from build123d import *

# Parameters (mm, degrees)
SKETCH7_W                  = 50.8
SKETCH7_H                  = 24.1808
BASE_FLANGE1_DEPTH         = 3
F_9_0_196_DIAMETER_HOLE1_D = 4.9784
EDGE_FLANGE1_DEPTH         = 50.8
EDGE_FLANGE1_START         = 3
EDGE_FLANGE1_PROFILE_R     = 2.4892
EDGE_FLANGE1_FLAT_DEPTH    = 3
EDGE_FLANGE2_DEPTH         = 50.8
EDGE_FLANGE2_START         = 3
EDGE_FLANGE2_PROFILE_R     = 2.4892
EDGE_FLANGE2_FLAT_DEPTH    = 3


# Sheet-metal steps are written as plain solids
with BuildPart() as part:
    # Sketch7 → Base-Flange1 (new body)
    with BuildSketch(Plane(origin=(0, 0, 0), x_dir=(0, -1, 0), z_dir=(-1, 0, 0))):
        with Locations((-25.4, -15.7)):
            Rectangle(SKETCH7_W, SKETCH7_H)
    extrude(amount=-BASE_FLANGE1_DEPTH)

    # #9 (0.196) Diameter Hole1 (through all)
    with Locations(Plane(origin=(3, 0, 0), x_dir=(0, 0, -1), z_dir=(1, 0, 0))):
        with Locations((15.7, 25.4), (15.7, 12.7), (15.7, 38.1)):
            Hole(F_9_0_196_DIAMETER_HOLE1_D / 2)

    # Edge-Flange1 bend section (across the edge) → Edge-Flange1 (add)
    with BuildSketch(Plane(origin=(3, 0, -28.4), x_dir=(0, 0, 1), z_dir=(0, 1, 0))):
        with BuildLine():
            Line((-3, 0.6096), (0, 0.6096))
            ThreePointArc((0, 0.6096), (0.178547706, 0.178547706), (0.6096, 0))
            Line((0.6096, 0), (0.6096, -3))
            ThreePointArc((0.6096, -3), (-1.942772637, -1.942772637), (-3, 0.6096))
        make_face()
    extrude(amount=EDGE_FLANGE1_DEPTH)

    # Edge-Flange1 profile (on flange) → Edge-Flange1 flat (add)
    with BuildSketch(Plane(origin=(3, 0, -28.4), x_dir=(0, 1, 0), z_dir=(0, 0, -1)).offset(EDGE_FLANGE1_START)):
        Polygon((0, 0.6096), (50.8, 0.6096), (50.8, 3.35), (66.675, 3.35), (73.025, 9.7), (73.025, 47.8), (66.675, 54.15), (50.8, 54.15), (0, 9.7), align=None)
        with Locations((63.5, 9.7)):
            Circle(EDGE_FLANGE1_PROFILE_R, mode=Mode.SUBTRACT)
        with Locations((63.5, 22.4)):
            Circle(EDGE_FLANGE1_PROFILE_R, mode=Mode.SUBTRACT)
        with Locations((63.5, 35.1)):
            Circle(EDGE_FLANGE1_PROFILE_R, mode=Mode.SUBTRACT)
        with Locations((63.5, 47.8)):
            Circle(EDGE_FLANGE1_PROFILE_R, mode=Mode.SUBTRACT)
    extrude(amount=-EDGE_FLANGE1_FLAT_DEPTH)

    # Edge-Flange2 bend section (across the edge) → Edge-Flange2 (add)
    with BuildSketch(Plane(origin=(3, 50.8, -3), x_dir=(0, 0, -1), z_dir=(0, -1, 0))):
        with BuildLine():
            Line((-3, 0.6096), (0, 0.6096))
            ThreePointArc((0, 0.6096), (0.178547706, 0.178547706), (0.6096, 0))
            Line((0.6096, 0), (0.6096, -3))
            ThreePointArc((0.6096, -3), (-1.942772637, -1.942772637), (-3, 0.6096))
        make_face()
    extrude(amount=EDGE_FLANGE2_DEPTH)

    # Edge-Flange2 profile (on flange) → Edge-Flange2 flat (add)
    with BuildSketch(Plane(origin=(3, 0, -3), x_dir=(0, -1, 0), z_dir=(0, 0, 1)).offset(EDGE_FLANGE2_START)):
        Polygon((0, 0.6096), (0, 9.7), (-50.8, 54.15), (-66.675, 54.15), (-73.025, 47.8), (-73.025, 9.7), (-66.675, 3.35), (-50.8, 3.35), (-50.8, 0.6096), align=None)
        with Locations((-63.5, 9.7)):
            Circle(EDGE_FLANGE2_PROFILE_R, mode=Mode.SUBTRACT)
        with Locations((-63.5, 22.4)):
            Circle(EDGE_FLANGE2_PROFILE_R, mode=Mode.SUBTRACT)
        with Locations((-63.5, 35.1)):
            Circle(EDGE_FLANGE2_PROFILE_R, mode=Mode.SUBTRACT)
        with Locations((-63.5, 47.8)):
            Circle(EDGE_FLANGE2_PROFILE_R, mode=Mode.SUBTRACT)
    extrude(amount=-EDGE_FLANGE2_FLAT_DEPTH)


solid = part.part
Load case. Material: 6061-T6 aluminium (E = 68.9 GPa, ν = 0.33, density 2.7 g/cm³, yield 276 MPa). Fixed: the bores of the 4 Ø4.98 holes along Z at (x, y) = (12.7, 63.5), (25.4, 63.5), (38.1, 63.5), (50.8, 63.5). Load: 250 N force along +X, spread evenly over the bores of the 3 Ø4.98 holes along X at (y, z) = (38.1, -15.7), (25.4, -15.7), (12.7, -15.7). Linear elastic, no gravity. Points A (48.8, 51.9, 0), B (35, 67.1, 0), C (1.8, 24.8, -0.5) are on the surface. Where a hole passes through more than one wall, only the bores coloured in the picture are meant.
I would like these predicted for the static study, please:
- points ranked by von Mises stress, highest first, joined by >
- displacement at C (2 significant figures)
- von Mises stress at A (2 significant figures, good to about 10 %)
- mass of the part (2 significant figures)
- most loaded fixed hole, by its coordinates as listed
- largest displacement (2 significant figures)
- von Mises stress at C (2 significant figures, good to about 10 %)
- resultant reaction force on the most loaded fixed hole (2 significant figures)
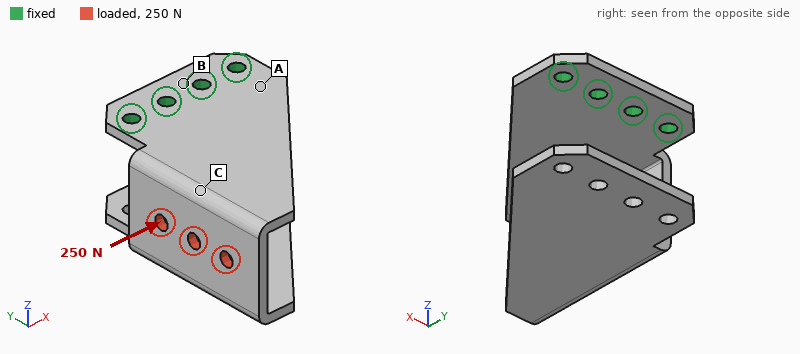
C > A > B
0.22 mm
16 MPa
54 g
(12.7, 63.5)
0.98 mm
28 MPa
280 N
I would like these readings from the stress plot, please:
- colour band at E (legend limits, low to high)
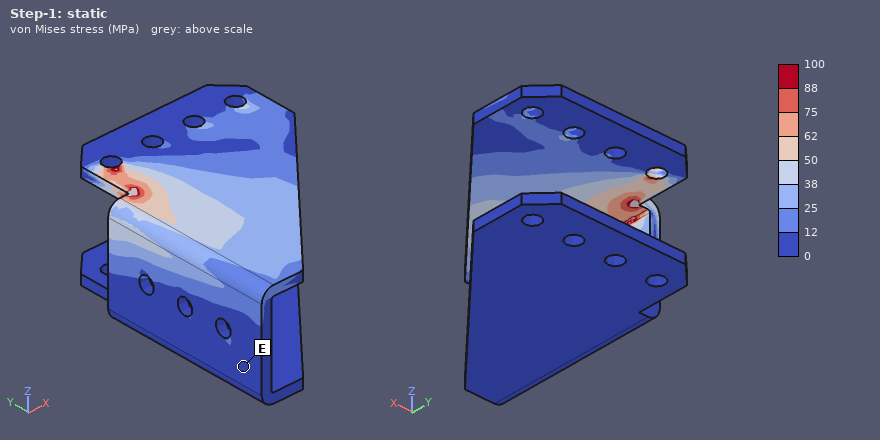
0 to 12 MPa
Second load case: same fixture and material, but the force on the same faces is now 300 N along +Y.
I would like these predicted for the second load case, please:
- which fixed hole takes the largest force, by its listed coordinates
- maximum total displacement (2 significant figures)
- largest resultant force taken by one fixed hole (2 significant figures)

(12.7, 63.5)
1.1 mm
320 N
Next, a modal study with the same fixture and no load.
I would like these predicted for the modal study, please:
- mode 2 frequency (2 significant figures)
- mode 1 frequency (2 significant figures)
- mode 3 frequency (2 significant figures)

380 Hz
320 Hz
730 Hz
